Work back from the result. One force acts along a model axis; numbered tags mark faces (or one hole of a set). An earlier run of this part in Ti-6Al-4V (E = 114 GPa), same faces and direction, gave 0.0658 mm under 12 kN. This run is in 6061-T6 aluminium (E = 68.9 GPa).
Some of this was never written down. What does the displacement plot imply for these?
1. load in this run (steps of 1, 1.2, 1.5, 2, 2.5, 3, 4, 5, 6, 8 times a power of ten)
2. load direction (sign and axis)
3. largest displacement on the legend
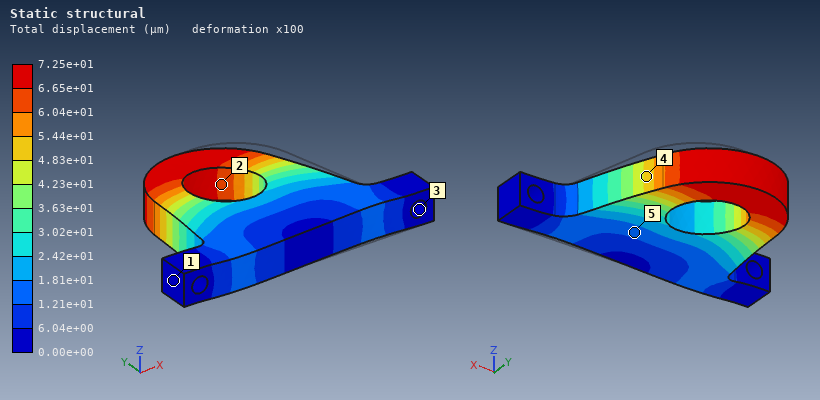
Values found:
8 kN
-X
7.25e+01 µm
